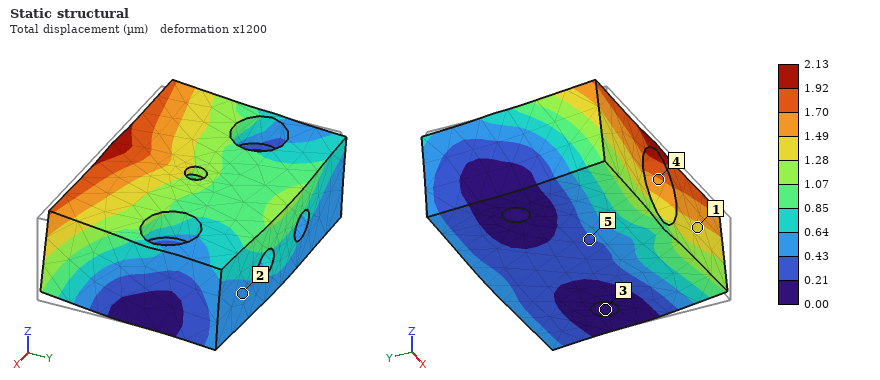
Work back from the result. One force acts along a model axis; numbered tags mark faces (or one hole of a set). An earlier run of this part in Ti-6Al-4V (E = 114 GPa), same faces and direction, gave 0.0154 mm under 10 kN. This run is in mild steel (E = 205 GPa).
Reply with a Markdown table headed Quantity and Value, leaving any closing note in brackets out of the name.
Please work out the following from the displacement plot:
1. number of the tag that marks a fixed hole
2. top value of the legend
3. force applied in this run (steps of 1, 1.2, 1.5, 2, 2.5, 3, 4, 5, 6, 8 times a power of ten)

| Quantity | Value |
|---|---|
| number of the tag that marks a fixed hole | 3 |
| top value of the legend | 2.13 µm |
| force applied in this run | 2.5 kN |
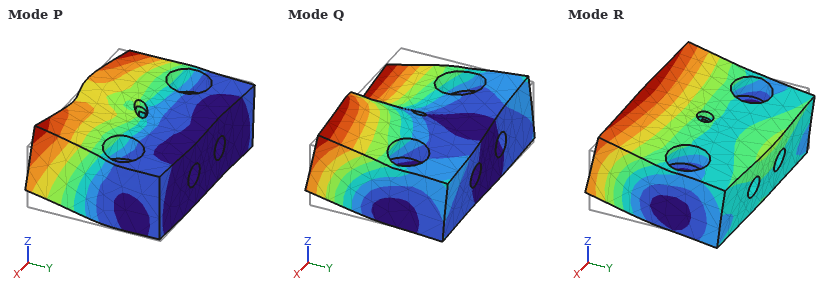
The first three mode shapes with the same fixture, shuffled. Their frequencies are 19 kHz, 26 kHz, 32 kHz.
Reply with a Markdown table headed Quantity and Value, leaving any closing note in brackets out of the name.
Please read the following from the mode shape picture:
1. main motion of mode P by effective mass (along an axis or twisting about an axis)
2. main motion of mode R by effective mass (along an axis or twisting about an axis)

| Quantity | Value |
|---|---|
| main motion of mode P by effective mass | along X |
| main motion of mode R by effective mass | along Z |
